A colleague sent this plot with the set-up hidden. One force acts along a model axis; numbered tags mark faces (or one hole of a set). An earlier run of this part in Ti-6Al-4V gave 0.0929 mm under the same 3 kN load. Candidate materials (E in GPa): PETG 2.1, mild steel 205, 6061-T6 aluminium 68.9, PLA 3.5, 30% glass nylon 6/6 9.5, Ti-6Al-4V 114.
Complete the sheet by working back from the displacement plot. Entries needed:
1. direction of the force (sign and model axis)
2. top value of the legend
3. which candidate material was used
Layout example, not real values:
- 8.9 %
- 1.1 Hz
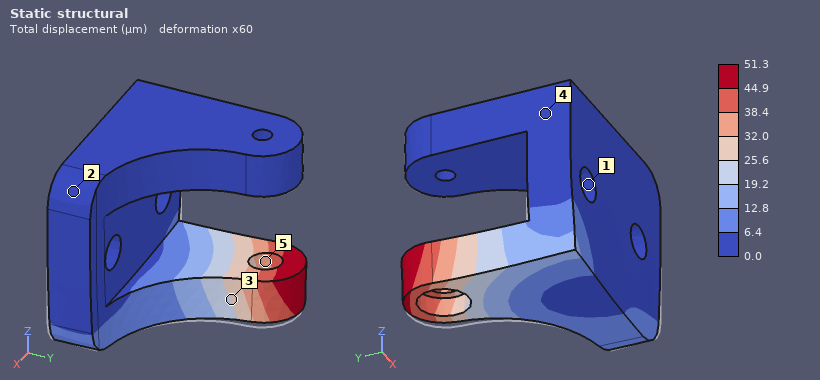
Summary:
- -X
- 51.3 µm
- mild steel
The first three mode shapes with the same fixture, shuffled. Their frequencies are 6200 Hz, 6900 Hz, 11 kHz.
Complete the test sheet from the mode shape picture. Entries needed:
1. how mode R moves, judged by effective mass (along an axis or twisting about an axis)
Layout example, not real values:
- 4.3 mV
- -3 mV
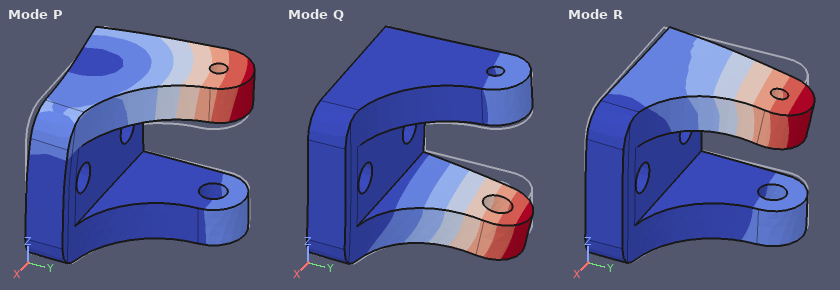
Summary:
- along Z
